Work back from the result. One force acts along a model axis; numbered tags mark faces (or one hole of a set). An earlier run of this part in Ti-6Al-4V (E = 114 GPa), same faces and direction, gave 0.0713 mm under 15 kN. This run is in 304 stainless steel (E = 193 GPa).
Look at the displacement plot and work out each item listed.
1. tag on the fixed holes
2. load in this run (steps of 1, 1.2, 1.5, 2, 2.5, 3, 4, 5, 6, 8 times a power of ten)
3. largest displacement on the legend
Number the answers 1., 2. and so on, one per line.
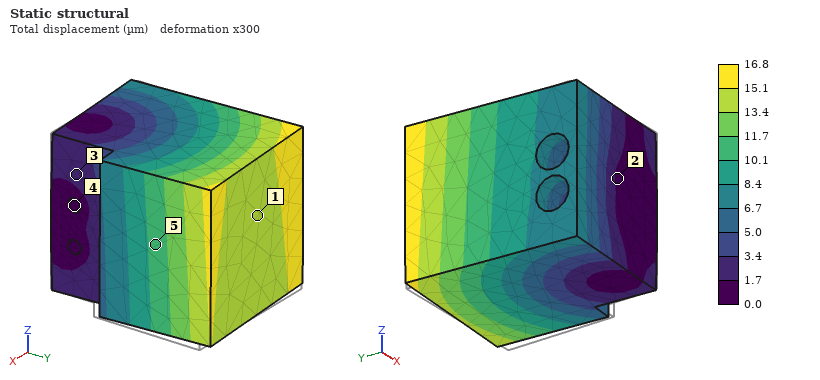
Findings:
1. 4
2. 6 kN
3. 16.8 µm
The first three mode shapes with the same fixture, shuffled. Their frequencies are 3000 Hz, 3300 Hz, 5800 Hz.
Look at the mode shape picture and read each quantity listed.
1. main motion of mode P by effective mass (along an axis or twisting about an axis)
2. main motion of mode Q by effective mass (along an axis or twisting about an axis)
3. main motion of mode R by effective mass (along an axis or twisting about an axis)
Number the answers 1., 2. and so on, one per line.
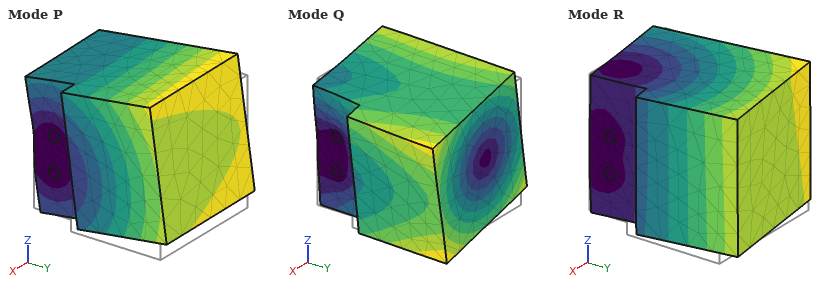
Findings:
1. along Z
2. twisting about Y
3. along X
